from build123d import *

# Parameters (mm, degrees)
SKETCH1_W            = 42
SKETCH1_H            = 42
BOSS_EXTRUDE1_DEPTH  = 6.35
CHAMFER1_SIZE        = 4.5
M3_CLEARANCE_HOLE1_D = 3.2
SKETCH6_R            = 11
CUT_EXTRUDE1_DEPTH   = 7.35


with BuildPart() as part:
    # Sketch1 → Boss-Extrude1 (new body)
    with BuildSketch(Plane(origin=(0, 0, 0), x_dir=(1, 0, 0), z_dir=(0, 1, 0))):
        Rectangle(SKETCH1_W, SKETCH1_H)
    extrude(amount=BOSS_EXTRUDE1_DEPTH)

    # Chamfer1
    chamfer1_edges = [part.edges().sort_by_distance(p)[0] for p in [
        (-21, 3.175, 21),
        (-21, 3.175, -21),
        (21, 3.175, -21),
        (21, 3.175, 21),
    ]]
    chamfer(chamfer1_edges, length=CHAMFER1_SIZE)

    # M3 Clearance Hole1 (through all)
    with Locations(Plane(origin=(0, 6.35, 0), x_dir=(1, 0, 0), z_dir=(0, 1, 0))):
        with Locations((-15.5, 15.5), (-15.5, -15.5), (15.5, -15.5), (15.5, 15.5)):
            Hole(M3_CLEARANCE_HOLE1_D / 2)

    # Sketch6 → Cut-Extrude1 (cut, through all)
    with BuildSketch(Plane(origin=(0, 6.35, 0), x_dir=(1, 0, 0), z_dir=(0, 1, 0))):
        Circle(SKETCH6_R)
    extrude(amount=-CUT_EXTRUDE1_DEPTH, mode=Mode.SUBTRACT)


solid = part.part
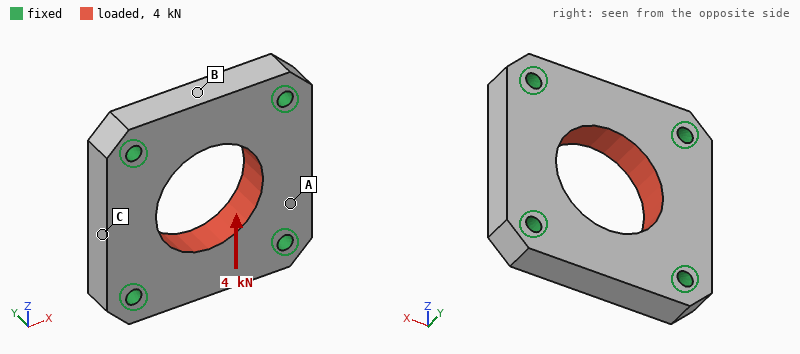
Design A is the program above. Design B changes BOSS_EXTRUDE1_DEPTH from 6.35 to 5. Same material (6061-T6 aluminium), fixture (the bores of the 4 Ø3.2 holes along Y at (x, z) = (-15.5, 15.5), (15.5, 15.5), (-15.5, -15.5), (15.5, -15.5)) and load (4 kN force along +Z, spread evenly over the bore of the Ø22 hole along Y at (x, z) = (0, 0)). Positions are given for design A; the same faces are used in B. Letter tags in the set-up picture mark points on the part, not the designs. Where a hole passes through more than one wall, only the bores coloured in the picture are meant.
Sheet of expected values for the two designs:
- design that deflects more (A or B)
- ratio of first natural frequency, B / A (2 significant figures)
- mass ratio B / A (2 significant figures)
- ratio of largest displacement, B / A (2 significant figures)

B
0.87
0.79
1.3
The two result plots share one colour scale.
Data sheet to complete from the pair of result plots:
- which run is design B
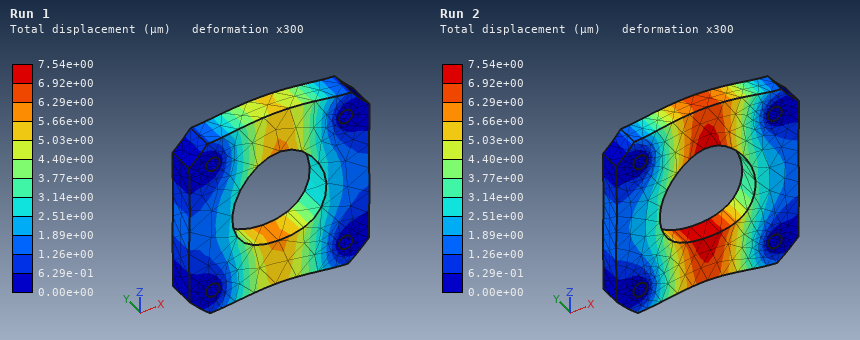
Run 2
